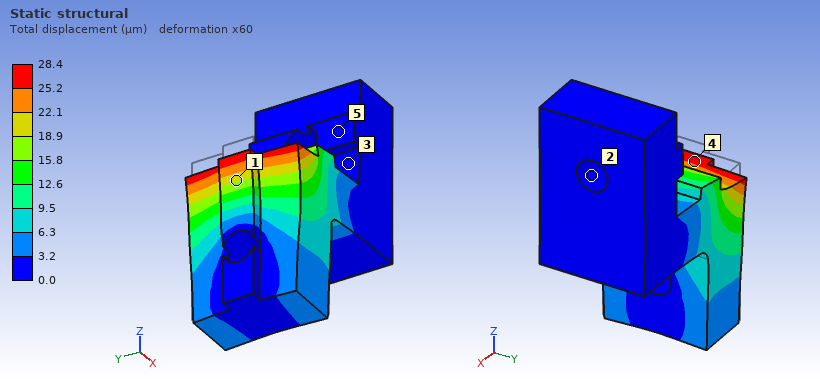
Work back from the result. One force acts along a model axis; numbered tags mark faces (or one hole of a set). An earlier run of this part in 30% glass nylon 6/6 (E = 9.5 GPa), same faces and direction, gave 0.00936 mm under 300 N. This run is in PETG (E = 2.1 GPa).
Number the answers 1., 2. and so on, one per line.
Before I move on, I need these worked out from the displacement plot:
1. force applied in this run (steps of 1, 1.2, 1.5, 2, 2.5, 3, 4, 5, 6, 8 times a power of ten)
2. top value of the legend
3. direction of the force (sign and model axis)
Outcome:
1. 200 N
2. 28.4 µm
3. -Z
